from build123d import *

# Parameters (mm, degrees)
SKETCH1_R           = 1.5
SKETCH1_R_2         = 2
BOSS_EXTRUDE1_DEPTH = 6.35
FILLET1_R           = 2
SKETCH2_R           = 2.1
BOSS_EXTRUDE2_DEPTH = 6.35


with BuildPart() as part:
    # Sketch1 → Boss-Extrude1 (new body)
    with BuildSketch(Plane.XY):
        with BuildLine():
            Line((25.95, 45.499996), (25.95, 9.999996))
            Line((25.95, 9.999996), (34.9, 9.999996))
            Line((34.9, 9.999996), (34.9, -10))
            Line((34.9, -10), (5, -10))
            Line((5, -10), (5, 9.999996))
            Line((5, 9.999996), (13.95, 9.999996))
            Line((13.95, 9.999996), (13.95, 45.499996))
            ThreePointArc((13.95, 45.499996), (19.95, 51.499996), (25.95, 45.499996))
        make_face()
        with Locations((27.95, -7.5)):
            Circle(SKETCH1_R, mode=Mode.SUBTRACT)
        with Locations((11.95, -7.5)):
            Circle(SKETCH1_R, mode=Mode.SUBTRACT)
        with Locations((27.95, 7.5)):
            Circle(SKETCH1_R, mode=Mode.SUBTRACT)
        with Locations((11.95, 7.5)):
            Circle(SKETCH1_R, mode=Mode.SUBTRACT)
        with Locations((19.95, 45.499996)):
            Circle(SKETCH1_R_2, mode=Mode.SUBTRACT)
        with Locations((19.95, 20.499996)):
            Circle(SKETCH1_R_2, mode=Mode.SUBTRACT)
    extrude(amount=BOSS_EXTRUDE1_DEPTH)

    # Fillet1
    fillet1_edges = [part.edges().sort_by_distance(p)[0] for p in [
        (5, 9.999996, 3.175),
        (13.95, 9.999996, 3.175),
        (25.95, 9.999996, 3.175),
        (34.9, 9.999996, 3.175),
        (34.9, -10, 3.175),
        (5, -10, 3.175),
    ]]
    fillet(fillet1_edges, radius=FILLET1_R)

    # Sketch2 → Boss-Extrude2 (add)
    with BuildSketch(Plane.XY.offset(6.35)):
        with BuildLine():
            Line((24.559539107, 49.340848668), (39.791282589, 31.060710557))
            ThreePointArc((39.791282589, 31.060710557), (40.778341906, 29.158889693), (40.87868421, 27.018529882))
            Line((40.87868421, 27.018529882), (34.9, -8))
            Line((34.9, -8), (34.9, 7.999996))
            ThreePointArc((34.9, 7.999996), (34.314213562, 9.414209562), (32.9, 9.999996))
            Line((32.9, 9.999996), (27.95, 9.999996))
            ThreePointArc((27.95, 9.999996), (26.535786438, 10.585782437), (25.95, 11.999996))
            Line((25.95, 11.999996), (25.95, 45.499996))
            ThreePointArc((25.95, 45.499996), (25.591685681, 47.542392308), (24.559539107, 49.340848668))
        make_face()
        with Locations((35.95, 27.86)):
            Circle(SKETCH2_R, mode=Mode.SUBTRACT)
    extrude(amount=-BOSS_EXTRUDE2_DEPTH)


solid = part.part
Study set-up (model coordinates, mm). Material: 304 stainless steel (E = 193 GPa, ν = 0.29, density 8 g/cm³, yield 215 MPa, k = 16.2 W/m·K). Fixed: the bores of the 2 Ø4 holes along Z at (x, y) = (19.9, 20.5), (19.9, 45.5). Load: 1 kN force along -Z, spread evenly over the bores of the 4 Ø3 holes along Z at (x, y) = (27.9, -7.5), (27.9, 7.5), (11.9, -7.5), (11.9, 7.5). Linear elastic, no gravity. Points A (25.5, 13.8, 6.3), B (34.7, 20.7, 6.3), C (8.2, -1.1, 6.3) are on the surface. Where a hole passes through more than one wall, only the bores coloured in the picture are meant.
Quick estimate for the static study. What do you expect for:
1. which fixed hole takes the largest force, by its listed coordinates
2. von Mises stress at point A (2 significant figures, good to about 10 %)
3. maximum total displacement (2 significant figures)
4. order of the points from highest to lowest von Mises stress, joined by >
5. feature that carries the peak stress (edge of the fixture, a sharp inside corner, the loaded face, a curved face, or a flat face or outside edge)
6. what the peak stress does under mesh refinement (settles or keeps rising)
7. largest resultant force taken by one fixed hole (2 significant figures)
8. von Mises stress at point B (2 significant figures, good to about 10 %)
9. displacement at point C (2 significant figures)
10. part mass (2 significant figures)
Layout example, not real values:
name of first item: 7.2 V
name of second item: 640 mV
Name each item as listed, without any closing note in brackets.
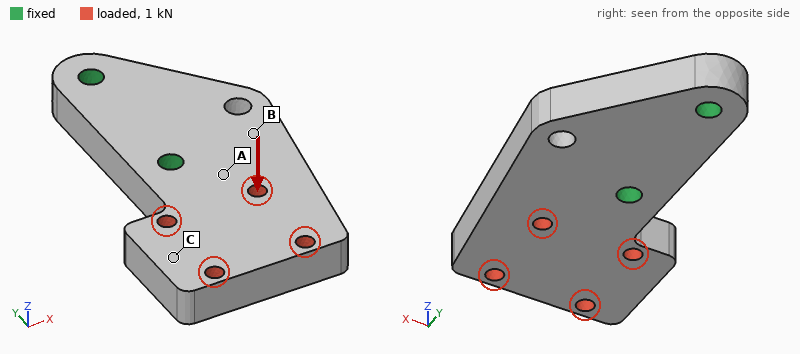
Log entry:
which fixed hole takes the largest force, by its listed coordinates: (19.9, 20.5)
von Mises stress at point A: 74 MPa
maximum total displacement: 69 µm
order of the points from highest to lowest von Mises stress, joined by >: A > B > C
feature that carries the peak stress: edge of the fixture
what the peak stress does under mesh refinement: keeps rising
largest resultant force taken by one fixed hole: 1.2 kN
von Mises stress at point B: 43 MPa
displacement at point C: 45 µm
part mass: 73 g
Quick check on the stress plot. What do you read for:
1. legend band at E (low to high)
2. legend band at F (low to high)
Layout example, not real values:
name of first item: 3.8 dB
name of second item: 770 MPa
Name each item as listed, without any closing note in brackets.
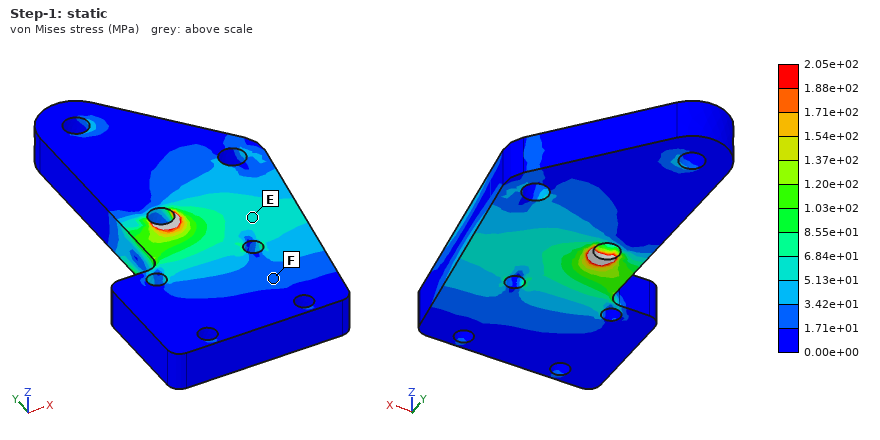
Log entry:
legend band at E: 5.13e+01 to 6.84e+01 MPa
legend band at F: 1.71e+01 to 3.42e+01 MPa
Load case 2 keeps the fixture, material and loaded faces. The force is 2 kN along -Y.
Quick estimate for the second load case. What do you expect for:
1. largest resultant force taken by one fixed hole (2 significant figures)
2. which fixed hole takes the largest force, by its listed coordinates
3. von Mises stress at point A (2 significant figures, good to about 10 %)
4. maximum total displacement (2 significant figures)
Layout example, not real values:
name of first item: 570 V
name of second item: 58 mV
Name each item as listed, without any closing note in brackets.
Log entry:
largest resultant force taken by one fixed hole: 1.8 kN
which fixed hole takes the largest force, by its listed coordinates: (19.9, 20.5)
von Mises stress at point A: 12 MPa
maximum total displacement: 5.7 µm
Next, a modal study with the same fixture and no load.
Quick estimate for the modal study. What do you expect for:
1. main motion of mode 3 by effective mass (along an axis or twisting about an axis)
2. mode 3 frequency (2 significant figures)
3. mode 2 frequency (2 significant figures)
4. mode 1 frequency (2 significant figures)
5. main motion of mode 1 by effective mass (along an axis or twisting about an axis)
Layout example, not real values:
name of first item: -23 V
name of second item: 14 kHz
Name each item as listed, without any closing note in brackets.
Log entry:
main motion of mode 3 by effective mass: along X
mode 3 frequency: 9200 Hz
mode 2 frequency: 7400 Hz
mode 1 frequency: 4400 Hz
main motion of mode 1 by effective mass: along Z
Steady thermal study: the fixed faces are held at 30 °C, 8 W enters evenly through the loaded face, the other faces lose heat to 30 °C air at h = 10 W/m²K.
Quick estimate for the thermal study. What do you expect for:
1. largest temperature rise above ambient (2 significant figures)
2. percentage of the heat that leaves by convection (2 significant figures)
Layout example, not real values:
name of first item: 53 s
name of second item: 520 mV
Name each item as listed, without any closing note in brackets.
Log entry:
largest temperature rise above ambient: 74 K
percentage of the heat that leaves by convection: 15 %
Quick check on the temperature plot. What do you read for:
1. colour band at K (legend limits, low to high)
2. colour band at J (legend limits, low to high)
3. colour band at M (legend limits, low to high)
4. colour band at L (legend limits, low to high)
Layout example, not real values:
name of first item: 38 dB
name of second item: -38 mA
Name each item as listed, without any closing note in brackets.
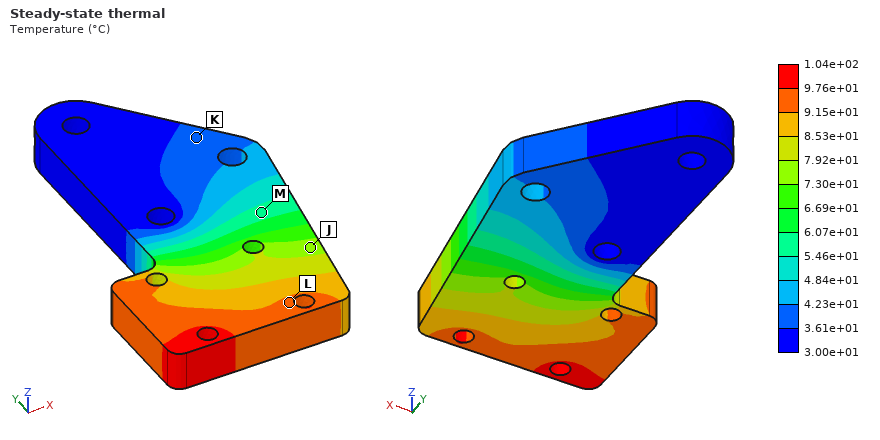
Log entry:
colour band at K: 3.61e+01 to 4.23e+01 °C
colour band at J: 7.30e+01 to 7.92e+01 °C
colour band at M: 5.46e+01 to 6.07e+01 °C
colour band at L: 9.15e+01 to 9.76e+01 °C
